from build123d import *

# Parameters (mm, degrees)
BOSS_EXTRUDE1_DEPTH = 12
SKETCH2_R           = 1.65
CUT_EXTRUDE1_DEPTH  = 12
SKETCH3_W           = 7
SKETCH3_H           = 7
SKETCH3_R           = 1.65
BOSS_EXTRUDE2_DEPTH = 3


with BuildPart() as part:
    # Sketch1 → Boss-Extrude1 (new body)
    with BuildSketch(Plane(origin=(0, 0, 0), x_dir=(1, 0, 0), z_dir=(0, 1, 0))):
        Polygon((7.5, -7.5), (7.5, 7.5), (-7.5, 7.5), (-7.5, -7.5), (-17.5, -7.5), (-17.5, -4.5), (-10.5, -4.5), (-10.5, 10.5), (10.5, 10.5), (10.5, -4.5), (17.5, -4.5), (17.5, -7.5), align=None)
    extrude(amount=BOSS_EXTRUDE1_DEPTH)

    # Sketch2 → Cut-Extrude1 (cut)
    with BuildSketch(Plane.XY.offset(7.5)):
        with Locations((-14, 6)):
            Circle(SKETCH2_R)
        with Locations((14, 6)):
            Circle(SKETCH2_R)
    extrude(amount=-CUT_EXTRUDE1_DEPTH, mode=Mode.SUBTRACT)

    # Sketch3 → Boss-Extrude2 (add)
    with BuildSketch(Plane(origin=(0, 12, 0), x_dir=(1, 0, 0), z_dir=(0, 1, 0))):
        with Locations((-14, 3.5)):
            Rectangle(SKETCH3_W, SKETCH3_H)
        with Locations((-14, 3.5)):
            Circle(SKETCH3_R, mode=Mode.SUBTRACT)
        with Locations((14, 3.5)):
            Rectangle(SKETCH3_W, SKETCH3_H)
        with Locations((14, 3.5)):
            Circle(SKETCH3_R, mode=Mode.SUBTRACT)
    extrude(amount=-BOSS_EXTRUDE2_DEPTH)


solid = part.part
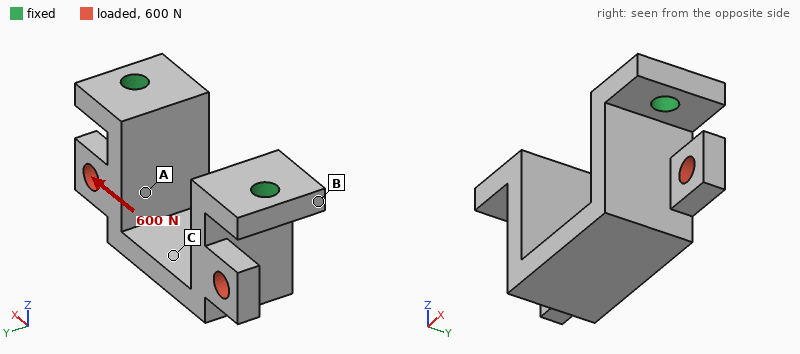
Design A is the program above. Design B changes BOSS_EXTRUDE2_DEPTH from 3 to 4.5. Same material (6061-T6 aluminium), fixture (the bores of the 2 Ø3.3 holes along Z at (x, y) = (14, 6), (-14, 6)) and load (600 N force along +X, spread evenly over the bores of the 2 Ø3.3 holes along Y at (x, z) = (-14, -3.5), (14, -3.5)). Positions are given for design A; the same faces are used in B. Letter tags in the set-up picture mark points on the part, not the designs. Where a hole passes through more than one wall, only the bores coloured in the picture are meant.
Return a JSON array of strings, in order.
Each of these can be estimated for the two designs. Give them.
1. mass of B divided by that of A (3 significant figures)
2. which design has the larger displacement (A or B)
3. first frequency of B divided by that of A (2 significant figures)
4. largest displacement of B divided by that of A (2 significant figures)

["1.05", "A", "0.98", "0.91"]
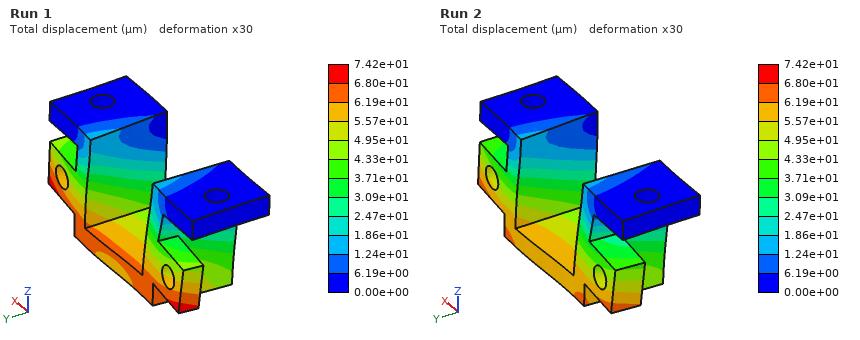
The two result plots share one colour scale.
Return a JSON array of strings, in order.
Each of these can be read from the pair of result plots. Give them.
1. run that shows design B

["Run 2"]
